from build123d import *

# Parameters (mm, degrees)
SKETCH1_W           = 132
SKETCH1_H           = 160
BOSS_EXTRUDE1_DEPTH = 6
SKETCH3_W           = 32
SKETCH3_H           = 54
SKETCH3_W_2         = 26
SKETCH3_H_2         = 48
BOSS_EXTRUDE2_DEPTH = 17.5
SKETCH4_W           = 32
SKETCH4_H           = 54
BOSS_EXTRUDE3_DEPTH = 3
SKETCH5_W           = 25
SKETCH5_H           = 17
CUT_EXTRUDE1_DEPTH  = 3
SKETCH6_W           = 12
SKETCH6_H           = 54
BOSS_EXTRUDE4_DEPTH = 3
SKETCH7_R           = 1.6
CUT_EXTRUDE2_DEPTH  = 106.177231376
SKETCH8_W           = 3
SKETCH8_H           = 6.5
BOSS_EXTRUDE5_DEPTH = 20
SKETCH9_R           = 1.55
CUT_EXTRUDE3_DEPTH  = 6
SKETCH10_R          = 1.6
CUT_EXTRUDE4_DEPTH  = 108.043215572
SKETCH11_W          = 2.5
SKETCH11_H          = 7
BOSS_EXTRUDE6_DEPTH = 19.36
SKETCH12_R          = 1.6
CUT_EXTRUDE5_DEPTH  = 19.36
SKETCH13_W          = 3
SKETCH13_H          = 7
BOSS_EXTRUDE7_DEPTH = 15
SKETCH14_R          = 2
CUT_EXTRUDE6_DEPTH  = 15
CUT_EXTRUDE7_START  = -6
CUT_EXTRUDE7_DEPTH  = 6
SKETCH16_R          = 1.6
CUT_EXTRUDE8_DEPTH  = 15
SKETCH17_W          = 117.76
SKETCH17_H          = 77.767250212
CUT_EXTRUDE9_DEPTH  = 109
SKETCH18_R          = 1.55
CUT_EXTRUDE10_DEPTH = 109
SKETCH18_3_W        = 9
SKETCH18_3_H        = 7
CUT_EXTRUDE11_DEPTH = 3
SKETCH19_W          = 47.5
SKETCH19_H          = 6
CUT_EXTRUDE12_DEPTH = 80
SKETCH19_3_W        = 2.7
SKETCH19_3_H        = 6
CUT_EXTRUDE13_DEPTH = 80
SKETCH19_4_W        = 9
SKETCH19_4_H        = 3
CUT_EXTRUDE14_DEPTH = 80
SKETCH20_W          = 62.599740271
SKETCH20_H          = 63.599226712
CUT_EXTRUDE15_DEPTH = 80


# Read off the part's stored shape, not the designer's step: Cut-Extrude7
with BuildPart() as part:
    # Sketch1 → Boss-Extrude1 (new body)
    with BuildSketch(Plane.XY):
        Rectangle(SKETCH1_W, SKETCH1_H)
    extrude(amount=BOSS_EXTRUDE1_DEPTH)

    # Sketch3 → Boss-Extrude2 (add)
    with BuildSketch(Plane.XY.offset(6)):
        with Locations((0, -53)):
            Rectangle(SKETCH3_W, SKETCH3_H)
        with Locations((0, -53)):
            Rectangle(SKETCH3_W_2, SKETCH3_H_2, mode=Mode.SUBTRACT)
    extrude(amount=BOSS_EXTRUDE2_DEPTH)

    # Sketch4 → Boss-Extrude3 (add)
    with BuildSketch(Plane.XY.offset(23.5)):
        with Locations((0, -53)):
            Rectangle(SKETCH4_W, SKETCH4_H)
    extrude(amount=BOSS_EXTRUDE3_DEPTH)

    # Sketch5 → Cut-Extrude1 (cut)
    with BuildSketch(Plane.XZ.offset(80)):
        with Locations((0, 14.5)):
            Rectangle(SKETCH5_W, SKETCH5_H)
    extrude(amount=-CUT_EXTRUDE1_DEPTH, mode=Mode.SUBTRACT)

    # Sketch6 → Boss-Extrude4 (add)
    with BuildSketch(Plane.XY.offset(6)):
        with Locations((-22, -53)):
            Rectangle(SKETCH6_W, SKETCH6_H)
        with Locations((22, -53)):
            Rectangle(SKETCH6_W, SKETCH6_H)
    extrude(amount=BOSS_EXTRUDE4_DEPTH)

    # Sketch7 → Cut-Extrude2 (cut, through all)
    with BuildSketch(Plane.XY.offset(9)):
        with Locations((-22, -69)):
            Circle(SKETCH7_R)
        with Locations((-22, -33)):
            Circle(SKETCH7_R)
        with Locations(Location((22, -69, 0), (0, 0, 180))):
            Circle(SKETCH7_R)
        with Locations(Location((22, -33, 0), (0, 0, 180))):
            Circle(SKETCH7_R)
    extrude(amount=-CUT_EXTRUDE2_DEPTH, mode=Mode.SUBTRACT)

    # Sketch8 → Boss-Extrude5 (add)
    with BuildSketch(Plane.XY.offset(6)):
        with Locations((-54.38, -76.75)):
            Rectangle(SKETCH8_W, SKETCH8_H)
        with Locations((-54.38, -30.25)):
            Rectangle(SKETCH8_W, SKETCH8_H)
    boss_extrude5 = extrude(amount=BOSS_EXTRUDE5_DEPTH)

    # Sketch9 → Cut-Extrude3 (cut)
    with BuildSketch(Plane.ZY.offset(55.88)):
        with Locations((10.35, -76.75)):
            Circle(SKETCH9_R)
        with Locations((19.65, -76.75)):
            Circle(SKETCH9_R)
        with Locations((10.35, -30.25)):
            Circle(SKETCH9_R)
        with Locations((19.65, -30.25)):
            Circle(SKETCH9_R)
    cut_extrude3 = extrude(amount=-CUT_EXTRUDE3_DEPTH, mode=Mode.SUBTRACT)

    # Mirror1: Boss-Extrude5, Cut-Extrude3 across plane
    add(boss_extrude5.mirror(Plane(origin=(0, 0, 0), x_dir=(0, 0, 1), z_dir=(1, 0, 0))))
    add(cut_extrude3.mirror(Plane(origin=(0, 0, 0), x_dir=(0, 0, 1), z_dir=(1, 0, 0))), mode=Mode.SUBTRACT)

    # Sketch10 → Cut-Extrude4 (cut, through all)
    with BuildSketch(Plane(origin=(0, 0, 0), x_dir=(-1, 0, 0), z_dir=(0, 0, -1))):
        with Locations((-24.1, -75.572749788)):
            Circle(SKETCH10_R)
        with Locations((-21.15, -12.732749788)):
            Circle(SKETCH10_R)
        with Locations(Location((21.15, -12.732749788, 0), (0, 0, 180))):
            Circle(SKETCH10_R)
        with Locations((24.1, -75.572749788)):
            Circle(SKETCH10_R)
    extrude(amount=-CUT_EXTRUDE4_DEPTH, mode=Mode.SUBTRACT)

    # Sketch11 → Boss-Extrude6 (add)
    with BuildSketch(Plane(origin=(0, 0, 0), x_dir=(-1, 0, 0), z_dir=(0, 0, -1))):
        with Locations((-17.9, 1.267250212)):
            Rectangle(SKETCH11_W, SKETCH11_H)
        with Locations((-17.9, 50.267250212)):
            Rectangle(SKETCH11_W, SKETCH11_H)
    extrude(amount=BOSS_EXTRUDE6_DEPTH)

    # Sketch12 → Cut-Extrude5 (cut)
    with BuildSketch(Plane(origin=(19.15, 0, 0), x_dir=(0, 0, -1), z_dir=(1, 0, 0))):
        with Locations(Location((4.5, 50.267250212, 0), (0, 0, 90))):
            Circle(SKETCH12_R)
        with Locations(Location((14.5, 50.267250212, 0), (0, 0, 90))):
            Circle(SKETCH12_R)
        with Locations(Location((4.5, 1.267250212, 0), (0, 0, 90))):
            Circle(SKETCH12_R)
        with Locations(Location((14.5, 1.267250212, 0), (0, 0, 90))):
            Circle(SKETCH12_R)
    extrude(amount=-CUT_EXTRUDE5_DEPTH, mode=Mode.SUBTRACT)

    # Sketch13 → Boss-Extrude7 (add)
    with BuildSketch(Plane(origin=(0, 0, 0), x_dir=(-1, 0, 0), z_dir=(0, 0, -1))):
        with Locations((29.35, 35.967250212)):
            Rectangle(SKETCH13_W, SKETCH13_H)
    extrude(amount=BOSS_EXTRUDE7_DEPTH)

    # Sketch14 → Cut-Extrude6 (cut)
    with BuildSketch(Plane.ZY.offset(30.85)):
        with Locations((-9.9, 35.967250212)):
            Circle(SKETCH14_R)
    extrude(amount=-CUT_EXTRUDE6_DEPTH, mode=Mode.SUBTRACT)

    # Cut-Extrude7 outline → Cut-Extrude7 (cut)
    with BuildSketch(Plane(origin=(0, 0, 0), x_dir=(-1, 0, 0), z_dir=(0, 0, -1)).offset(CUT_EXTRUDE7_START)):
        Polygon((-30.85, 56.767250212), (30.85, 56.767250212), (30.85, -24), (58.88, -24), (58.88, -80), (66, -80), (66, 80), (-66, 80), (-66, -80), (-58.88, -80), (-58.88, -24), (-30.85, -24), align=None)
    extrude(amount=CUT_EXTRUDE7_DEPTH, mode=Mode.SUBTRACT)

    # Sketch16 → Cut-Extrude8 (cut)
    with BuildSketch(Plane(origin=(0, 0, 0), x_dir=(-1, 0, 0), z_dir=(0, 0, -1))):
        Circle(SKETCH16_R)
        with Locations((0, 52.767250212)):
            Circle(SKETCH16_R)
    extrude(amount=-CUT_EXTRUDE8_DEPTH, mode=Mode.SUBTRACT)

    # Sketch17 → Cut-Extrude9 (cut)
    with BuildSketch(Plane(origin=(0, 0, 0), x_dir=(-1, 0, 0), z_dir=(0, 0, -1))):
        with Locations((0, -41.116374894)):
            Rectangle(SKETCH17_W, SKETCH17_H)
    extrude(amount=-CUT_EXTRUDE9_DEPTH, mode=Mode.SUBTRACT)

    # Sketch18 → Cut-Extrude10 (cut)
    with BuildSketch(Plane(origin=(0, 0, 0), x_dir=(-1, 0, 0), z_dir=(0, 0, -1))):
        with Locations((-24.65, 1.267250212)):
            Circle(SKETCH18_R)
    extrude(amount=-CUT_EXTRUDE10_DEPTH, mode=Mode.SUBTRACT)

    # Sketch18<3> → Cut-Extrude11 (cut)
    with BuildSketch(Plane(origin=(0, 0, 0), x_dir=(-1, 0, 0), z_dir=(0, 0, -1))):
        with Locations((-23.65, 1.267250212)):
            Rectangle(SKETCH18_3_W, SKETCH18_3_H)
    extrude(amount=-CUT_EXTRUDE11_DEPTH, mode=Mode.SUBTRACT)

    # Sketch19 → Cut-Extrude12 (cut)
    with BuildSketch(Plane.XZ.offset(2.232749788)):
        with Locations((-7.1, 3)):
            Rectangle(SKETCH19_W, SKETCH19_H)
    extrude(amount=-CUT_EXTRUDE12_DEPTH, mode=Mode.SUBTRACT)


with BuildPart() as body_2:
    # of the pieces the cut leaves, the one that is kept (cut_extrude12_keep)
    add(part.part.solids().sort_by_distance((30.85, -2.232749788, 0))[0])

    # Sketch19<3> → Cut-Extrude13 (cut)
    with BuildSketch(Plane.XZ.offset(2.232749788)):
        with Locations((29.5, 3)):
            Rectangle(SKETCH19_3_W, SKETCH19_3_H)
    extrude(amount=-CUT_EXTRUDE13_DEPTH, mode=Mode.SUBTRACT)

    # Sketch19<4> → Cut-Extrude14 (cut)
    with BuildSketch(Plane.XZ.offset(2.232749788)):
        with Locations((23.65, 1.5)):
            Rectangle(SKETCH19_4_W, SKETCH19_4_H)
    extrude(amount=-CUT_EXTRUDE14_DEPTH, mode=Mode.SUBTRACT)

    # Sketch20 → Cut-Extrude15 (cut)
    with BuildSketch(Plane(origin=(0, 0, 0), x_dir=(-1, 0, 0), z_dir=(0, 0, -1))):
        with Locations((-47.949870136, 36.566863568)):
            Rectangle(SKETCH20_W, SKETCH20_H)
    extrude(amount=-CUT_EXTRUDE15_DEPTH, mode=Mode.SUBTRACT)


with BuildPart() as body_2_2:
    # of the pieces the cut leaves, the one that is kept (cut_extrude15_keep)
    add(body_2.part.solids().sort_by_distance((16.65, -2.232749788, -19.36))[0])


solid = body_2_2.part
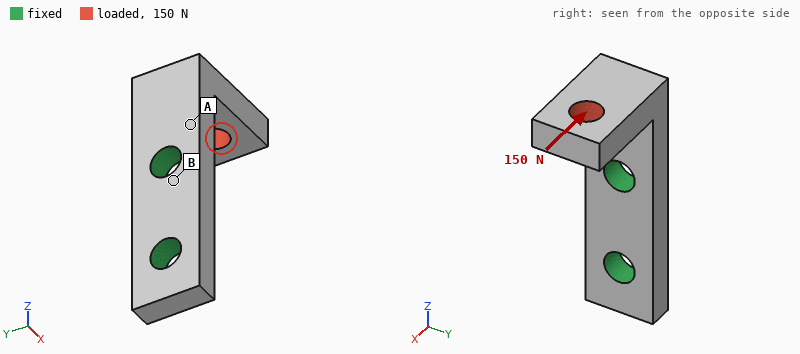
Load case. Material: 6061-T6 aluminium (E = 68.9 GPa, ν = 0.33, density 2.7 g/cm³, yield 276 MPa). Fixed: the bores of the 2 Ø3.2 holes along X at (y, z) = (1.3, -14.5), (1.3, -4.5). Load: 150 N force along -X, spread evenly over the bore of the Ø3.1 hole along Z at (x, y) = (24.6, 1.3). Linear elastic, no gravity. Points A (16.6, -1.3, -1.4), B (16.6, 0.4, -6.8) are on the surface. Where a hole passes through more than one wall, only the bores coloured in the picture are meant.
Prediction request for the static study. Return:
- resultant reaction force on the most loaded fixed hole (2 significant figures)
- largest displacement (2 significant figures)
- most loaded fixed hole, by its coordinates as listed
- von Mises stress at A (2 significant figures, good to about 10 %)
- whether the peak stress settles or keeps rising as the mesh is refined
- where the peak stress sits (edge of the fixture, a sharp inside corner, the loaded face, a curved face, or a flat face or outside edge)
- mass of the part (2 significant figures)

150 N
95 µm
(1.3, -4.5)
100 MPa
keeps rising
edge of the fixture
1.5 g
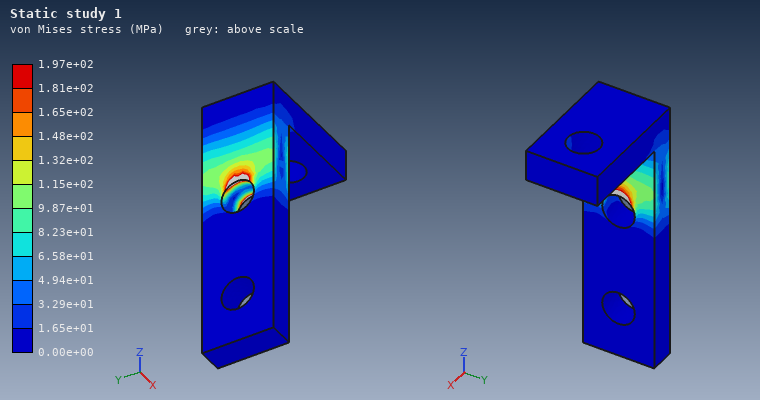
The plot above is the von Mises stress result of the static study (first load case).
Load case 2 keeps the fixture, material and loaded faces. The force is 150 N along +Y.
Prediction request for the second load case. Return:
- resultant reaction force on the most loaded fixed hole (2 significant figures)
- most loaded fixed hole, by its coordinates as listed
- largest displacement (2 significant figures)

180 N
(1.3, -4.5)
0.11 mm
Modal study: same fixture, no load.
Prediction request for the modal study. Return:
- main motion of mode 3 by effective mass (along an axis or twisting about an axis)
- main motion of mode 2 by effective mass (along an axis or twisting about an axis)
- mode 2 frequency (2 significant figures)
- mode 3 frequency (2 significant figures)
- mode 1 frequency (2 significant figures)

along X
along Y
11 kHz
24 kHz
8100 Hz
